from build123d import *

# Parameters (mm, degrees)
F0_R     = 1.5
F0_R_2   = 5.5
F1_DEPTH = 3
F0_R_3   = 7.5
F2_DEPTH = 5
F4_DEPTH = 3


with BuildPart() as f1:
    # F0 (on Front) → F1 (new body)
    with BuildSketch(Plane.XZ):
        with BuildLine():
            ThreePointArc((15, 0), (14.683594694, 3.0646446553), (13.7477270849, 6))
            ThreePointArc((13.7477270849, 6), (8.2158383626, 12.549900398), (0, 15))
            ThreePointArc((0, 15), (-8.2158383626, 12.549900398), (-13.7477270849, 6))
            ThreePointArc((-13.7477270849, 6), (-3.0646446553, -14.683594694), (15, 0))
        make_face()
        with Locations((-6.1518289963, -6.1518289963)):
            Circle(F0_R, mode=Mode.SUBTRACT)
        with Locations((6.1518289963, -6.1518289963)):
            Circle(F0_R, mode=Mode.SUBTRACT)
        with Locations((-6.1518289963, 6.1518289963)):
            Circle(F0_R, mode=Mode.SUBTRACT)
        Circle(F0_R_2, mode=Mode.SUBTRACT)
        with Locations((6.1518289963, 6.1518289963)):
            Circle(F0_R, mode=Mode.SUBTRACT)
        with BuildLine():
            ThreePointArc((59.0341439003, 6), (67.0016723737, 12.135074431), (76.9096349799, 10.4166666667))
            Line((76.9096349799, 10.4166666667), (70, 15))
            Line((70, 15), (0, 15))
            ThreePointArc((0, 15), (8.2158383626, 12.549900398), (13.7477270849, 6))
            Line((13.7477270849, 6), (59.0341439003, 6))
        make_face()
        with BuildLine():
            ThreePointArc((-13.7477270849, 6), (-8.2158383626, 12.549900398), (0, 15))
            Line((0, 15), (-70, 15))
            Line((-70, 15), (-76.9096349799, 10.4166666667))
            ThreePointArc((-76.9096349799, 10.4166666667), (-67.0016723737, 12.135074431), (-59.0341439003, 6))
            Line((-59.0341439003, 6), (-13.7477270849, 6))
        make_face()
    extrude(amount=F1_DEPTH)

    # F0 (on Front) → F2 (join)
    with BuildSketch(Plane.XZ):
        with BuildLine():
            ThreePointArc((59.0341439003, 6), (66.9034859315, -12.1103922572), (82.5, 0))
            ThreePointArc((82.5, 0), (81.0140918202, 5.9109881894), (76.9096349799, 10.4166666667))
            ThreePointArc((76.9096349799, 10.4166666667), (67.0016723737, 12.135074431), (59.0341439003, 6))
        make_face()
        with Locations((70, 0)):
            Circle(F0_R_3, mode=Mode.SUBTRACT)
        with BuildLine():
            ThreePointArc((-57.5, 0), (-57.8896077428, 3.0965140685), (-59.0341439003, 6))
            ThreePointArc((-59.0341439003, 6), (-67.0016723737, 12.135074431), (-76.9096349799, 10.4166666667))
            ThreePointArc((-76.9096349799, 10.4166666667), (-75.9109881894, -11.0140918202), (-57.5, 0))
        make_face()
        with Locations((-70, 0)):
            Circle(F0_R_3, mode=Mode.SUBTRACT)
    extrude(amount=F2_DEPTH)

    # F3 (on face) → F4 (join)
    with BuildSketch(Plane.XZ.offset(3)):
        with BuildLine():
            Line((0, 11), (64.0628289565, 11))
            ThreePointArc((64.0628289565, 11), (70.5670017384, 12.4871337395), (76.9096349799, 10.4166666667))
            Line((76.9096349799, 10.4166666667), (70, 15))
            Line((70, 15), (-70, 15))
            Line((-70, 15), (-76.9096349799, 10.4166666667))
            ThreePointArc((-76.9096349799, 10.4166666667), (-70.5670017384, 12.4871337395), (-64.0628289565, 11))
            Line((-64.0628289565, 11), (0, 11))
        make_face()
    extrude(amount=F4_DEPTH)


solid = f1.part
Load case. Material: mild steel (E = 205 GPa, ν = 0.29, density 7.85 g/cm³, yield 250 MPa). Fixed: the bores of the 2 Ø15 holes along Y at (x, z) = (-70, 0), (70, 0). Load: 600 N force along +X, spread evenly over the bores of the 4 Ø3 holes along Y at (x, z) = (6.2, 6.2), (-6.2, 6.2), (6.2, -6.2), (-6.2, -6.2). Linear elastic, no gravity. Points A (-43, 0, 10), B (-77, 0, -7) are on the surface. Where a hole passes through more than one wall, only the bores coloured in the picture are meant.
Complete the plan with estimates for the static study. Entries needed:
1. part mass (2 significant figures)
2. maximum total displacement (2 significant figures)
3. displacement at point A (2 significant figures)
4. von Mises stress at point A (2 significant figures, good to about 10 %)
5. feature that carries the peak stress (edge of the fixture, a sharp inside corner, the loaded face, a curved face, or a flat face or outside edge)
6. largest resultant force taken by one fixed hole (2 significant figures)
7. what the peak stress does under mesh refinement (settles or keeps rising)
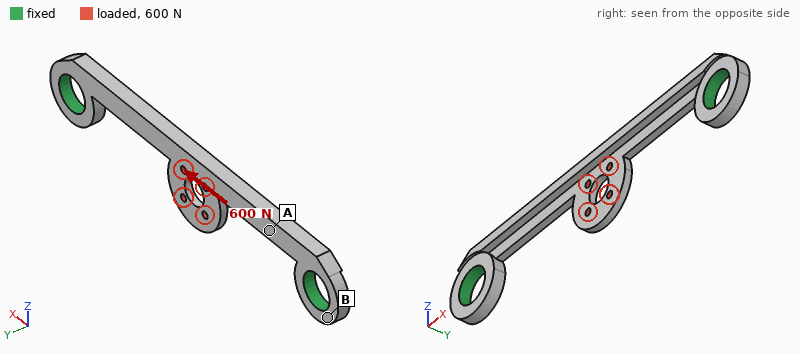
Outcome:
75 g
22 µm
6.2 µm
12 MPa
a sharp inside corner
310 N
keeps rising
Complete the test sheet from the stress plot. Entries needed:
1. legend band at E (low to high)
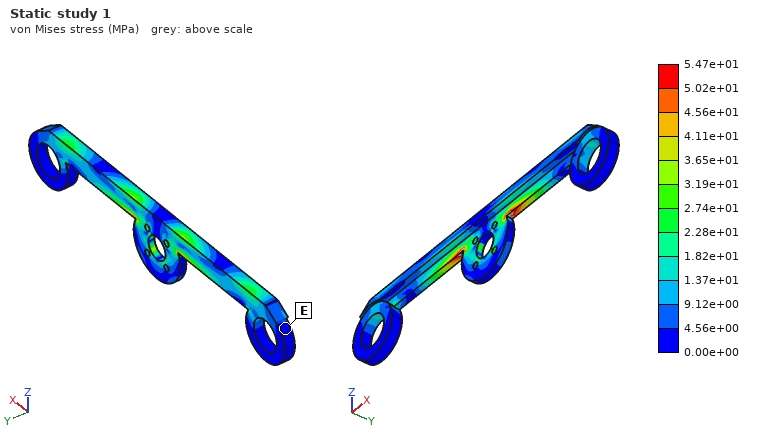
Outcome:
0.00e+00 to 4.56e+00 MPa
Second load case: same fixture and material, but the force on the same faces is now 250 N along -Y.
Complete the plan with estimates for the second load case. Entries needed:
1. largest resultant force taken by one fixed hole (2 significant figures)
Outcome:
130 N
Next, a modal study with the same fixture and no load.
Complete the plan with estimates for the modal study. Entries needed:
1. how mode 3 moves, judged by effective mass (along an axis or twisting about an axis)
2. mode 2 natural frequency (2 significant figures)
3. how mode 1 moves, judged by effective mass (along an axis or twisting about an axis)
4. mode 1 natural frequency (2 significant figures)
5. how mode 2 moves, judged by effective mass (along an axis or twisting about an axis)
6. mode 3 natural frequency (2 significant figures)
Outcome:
along Z
2100 Hz
along Y
1100 Hz
along Z
2600 Hz
